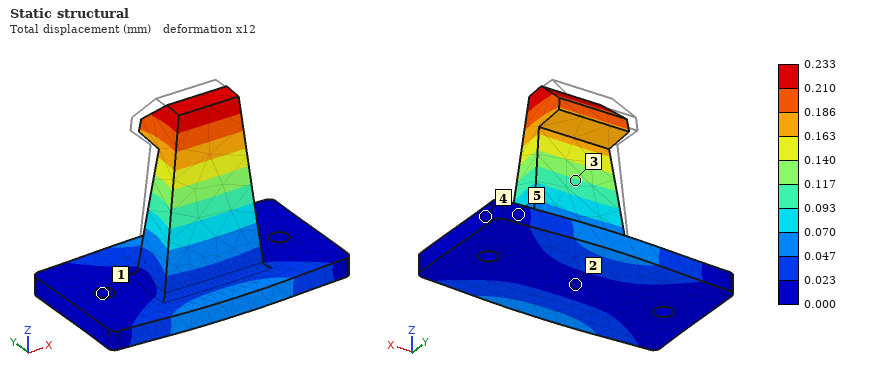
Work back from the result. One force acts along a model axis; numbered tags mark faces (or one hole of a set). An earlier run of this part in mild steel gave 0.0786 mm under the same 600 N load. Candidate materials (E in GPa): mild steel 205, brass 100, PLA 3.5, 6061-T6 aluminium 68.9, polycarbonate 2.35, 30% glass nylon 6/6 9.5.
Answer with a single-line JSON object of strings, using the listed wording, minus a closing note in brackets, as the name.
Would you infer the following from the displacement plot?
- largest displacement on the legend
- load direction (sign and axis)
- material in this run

{"largest displacement on the legend": "0.233 mm", "load direction": "-Y", "material in this run": "6061-T6 aluminium"}
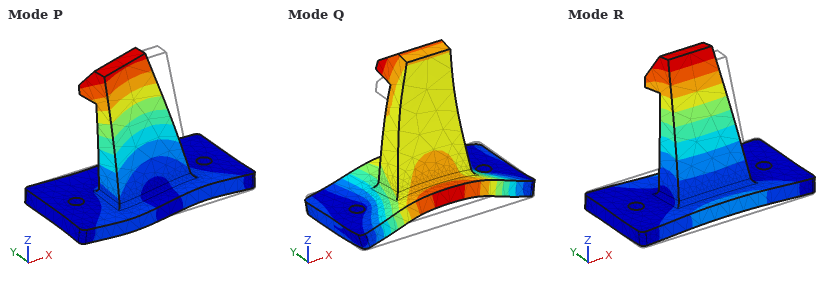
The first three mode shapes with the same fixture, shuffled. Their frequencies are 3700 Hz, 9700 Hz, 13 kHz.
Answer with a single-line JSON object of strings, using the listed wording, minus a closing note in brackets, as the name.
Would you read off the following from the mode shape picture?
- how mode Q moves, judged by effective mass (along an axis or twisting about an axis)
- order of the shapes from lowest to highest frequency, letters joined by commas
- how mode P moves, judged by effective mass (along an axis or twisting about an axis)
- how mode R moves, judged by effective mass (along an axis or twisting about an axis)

{"how mode Q moves, judged by effective mass": "along Z", "order of the shapes from lowest to highest frequency, letters joined by commas": "R, P, Q", "how mode P moves, judged by effective mass": "along X", "how mode R moves, judged by effective mass": "along Y"}
